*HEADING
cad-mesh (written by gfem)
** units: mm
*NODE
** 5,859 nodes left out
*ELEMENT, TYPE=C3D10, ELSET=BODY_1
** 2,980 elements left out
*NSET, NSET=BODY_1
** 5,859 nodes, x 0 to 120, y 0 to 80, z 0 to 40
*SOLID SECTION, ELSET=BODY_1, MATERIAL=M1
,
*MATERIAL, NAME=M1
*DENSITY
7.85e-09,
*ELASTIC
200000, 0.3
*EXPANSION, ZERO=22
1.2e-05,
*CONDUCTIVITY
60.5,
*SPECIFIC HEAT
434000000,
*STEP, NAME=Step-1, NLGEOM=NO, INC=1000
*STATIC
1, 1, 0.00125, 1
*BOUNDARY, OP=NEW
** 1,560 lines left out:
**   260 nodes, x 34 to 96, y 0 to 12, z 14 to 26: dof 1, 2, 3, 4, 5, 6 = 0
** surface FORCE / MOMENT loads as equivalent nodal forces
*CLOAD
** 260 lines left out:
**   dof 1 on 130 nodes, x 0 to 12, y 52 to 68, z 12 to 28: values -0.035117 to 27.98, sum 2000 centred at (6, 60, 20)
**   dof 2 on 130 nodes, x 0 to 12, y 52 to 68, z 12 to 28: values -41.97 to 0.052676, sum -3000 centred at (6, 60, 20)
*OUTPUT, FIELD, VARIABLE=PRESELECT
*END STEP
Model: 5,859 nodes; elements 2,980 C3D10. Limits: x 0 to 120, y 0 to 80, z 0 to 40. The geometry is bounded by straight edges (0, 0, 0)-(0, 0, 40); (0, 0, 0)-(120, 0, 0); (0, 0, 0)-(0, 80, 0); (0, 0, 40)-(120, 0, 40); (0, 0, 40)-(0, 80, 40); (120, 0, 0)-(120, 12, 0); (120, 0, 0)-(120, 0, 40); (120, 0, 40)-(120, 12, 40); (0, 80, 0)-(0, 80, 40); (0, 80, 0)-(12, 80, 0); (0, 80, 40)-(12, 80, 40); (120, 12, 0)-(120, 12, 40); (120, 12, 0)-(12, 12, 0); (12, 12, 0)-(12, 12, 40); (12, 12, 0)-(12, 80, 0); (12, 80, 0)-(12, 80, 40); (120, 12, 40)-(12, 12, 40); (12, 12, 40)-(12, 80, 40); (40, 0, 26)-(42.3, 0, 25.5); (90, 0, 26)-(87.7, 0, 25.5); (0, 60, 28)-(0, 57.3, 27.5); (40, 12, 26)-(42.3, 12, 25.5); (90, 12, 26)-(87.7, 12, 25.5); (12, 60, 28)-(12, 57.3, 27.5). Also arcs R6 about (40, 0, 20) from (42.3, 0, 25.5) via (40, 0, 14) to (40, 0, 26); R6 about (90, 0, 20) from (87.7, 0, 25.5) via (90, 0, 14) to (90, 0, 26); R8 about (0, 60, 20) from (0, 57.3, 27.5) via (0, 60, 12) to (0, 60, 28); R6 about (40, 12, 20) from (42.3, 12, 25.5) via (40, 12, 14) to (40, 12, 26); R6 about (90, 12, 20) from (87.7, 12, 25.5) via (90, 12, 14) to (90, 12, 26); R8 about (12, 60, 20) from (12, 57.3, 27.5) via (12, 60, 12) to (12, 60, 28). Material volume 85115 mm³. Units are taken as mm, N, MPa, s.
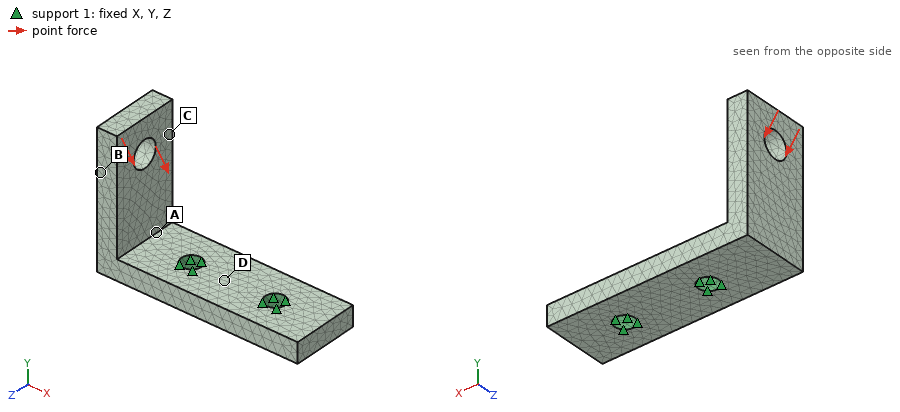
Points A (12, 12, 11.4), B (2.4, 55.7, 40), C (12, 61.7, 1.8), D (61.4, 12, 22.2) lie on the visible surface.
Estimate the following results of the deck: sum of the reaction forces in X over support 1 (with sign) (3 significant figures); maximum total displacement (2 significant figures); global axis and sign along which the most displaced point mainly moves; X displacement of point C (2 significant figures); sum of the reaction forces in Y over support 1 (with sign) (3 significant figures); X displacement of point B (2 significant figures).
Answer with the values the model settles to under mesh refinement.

-2000 N
0.24 mm
+X
0.16 mm
3000 N
0.14 mm
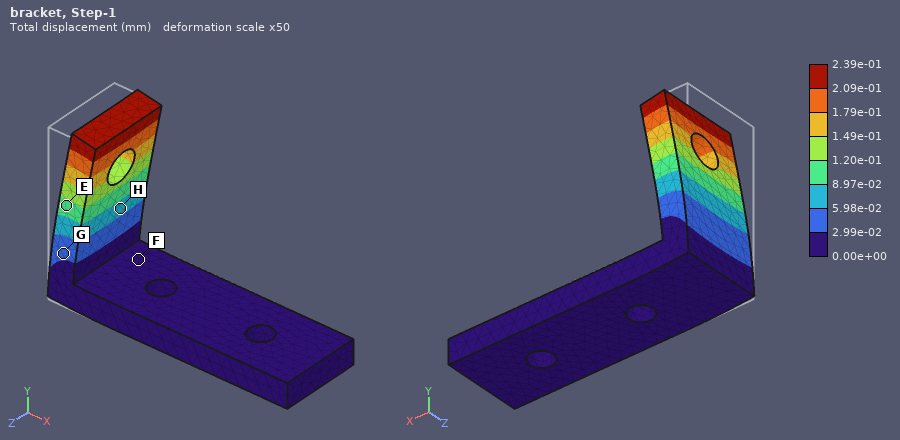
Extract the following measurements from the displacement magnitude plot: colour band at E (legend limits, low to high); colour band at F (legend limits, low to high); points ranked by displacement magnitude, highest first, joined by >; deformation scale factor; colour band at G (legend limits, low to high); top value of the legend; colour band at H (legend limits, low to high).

8.97e-02 to 1.20e-01 mm
0.00e+00 to 2.99e-02 mm
E > H > G > F
50
2.99e-02 to 5.98e-02 mm
2.39e-01 mm
5.98e-02 to 8.97e-02 mm
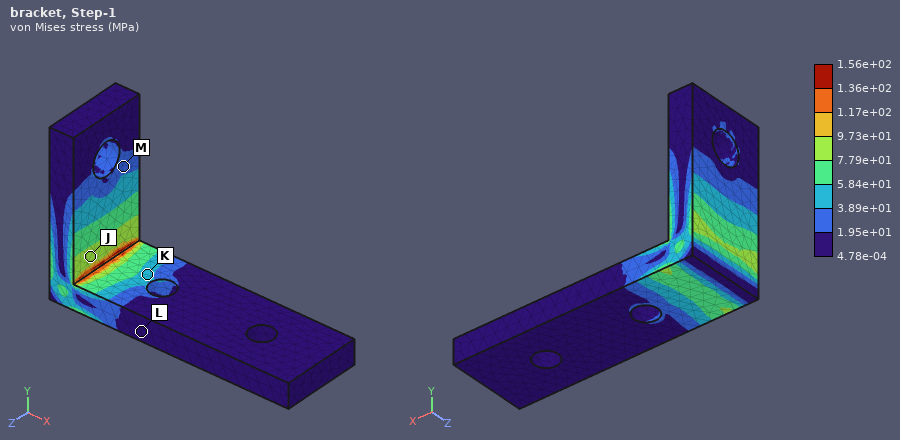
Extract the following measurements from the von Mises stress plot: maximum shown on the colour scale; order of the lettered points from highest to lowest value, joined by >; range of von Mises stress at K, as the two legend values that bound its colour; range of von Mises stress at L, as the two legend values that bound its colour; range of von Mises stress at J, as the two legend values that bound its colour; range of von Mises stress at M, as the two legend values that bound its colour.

1.56e+02 MPa
J > K > M > L
3.89e+01 to 5.84e+01 MPa
4.78e-04 to 1.95e+01 MPa
7.79e+01 to 9.73e+01 MPa
1.95e+01 to 3.89e+01 MPa
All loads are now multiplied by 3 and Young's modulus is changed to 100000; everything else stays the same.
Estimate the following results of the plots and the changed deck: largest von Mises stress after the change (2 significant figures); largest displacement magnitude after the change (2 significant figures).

470 MPa
1.4 mm
